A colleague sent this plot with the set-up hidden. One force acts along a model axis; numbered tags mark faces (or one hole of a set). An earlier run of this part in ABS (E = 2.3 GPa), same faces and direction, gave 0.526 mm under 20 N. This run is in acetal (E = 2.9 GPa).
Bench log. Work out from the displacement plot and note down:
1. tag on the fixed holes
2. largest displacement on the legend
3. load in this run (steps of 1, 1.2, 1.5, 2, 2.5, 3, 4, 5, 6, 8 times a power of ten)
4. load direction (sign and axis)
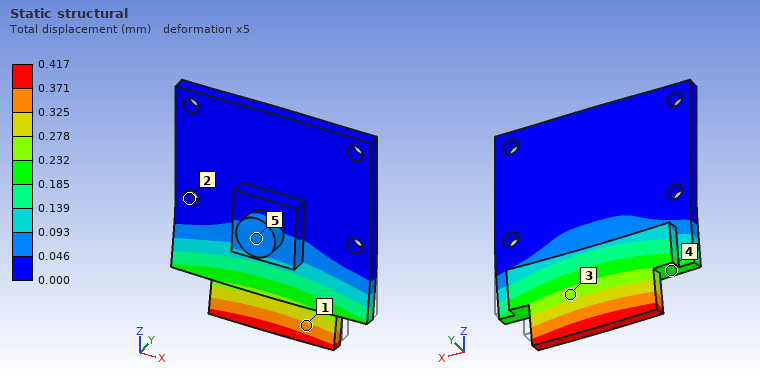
2
0.417 mm
20 N
-Y
